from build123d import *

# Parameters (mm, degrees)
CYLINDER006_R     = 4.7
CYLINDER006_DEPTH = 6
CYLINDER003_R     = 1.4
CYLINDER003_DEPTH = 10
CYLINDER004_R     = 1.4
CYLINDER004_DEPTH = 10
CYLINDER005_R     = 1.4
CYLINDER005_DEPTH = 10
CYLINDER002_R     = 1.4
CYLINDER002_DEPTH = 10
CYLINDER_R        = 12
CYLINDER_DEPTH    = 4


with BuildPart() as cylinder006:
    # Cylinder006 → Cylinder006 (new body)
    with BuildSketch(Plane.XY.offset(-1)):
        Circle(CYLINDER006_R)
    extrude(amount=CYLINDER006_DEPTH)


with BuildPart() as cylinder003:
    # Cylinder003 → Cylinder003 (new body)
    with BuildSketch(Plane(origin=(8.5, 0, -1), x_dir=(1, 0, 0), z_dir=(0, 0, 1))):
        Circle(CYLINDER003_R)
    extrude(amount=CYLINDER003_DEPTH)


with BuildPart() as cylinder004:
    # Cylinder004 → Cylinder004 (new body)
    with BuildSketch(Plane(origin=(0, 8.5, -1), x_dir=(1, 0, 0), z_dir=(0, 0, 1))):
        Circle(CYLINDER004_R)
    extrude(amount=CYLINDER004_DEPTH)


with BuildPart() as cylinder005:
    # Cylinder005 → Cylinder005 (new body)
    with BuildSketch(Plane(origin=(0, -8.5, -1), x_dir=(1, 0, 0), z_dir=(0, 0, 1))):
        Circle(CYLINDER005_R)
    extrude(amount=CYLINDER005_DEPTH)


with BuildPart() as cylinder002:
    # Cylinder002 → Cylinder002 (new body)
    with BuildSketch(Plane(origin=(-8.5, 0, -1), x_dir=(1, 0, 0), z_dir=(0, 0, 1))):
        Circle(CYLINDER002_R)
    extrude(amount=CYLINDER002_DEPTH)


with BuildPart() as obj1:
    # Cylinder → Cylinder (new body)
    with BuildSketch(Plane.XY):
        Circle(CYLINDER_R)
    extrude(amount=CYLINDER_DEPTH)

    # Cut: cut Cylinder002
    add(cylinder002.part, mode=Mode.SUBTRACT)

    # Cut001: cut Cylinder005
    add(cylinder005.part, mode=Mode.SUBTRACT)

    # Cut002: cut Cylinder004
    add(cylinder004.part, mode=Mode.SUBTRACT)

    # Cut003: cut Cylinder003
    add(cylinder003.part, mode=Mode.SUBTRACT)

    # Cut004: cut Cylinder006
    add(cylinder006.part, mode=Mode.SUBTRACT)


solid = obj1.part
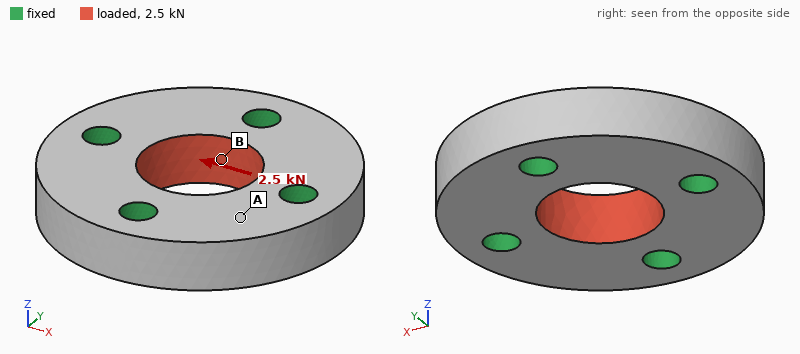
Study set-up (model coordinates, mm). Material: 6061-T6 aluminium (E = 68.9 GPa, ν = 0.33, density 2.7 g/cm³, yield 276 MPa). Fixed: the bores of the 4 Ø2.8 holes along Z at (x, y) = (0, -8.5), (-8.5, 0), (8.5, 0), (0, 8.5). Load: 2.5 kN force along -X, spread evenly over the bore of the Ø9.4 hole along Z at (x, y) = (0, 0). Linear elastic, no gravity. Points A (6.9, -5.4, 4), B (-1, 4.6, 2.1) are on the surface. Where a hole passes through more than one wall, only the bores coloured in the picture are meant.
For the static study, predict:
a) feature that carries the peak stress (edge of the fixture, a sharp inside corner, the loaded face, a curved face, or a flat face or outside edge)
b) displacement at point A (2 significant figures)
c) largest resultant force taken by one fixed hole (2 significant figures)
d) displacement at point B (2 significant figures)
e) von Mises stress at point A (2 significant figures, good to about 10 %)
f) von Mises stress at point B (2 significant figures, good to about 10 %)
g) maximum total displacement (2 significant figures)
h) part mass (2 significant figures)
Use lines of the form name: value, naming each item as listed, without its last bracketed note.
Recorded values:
feature that carries the peak stress: edge of the fixture
displacement at point A: 1.3 µm
largest resultant force taken by one fixed hole: 690 N
displacement at point B: 2.3 µm
von Mises stress at point A: 9.1 MPa
von Mises stress at point B: 36 MPa
maximum total displacement: 2.3 µm
part mass: 3.9 g
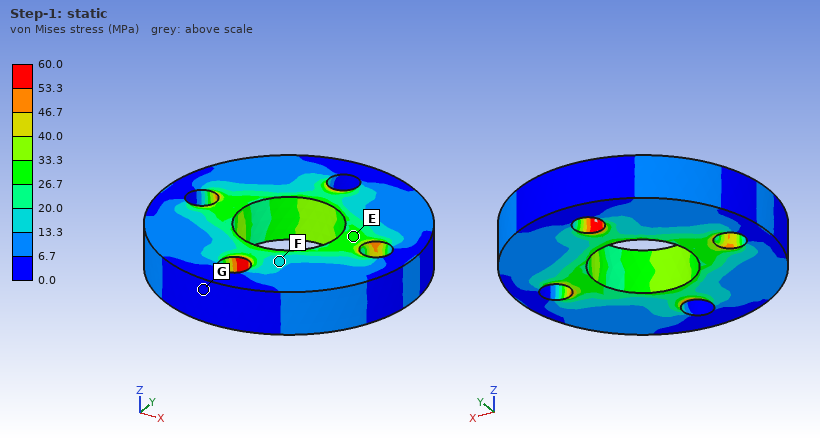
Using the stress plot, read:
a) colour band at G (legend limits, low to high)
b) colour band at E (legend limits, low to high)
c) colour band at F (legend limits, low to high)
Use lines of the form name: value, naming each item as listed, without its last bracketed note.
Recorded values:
colour band at G: 0.0 to 6.7 MPa
colour band at E: 26.7 to 33.3 MPa
colour band at F: 13.3 to 20.0 MPa
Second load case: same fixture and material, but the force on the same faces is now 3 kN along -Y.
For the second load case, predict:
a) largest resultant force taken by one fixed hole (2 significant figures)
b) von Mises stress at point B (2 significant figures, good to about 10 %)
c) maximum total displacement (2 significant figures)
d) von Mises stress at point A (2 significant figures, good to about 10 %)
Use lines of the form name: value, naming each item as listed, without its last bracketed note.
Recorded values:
largest resultant force taken by one fixed hole: 820 N
von Mises stress at point B: 35 MPa
maximum total displacement: 2.8 µm
von Mises stress at point A: 12 MPa
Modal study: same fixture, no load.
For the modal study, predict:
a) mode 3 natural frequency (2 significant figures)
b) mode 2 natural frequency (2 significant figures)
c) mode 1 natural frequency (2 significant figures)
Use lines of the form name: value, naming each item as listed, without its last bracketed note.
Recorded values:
mode 3 natural frequency: 74 kHz
mode 2 natural frequency: 74 kHz
mode 1 natural frequency: 72 kHz
